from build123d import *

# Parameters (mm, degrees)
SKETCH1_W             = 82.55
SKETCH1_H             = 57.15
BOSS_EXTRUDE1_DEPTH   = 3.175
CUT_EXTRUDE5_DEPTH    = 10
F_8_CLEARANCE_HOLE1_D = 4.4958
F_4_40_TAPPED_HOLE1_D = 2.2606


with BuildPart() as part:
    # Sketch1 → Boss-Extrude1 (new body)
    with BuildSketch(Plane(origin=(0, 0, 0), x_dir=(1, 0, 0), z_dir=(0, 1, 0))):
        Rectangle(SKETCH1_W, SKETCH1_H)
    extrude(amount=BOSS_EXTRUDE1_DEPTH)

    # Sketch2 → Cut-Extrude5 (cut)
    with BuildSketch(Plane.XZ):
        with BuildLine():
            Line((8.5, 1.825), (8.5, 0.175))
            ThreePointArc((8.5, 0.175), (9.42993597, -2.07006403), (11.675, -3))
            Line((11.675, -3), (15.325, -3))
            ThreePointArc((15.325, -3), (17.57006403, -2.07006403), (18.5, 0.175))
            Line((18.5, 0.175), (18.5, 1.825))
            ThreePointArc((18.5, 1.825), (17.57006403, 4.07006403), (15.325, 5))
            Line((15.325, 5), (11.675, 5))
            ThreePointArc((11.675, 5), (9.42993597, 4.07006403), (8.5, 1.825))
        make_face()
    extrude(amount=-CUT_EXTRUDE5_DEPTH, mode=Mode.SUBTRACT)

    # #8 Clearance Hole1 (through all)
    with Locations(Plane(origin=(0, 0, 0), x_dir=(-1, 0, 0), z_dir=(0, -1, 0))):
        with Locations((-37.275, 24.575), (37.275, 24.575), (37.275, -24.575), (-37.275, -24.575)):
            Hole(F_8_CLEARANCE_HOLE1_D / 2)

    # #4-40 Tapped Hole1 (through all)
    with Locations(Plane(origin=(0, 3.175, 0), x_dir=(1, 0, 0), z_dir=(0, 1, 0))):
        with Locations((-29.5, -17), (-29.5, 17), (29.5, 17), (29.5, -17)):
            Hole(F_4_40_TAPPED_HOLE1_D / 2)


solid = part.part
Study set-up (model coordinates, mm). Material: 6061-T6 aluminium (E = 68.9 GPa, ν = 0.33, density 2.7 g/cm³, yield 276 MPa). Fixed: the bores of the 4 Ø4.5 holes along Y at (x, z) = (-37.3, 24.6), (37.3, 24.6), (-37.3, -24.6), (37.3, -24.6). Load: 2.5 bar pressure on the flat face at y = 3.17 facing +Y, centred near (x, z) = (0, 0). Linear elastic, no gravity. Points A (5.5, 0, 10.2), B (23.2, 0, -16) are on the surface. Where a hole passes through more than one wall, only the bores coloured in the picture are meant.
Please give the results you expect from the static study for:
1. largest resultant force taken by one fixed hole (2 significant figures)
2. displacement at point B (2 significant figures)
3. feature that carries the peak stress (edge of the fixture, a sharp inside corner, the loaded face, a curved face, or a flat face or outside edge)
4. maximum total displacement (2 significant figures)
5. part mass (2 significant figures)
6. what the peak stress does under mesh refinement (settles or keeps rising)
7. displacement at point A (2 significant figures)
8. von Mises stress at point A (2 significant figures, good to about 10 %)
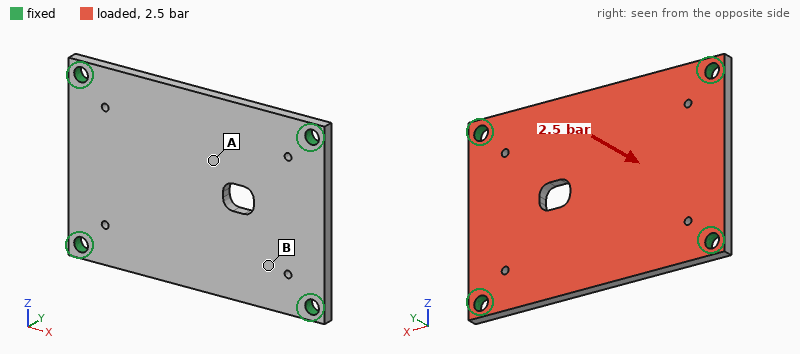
290 N
0.072 mm
edge of the fixture
0.16 mm
39 g
keeps rising
0.15 mm
35 MPa
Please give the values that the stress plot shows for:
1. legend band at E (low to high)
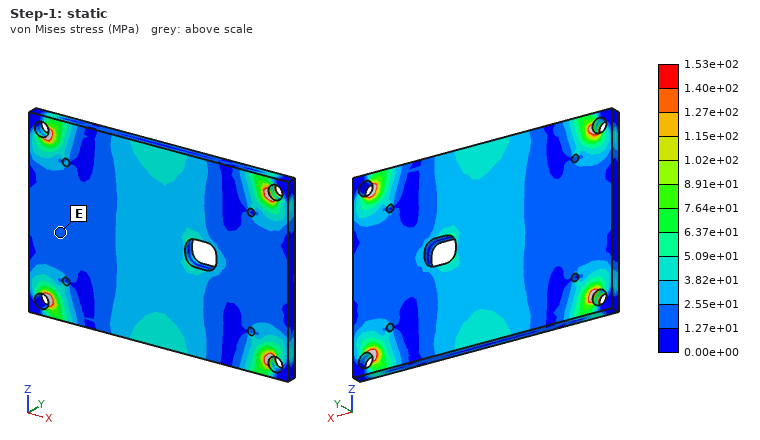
1.27e+01 to 2.55e+01 MPa
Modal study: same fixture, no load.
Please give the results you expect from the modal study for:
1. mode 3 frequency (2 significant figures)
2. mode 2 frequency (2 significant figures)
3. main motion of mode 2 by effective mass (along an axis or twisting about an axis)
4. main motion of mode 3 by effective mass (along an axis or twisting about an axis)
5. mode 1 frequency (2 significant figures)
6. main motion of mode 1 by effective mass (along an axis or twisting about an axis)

6100 Hz
4000 Hz
twisting about X
twisting about Z
2500 Hz
along Y
